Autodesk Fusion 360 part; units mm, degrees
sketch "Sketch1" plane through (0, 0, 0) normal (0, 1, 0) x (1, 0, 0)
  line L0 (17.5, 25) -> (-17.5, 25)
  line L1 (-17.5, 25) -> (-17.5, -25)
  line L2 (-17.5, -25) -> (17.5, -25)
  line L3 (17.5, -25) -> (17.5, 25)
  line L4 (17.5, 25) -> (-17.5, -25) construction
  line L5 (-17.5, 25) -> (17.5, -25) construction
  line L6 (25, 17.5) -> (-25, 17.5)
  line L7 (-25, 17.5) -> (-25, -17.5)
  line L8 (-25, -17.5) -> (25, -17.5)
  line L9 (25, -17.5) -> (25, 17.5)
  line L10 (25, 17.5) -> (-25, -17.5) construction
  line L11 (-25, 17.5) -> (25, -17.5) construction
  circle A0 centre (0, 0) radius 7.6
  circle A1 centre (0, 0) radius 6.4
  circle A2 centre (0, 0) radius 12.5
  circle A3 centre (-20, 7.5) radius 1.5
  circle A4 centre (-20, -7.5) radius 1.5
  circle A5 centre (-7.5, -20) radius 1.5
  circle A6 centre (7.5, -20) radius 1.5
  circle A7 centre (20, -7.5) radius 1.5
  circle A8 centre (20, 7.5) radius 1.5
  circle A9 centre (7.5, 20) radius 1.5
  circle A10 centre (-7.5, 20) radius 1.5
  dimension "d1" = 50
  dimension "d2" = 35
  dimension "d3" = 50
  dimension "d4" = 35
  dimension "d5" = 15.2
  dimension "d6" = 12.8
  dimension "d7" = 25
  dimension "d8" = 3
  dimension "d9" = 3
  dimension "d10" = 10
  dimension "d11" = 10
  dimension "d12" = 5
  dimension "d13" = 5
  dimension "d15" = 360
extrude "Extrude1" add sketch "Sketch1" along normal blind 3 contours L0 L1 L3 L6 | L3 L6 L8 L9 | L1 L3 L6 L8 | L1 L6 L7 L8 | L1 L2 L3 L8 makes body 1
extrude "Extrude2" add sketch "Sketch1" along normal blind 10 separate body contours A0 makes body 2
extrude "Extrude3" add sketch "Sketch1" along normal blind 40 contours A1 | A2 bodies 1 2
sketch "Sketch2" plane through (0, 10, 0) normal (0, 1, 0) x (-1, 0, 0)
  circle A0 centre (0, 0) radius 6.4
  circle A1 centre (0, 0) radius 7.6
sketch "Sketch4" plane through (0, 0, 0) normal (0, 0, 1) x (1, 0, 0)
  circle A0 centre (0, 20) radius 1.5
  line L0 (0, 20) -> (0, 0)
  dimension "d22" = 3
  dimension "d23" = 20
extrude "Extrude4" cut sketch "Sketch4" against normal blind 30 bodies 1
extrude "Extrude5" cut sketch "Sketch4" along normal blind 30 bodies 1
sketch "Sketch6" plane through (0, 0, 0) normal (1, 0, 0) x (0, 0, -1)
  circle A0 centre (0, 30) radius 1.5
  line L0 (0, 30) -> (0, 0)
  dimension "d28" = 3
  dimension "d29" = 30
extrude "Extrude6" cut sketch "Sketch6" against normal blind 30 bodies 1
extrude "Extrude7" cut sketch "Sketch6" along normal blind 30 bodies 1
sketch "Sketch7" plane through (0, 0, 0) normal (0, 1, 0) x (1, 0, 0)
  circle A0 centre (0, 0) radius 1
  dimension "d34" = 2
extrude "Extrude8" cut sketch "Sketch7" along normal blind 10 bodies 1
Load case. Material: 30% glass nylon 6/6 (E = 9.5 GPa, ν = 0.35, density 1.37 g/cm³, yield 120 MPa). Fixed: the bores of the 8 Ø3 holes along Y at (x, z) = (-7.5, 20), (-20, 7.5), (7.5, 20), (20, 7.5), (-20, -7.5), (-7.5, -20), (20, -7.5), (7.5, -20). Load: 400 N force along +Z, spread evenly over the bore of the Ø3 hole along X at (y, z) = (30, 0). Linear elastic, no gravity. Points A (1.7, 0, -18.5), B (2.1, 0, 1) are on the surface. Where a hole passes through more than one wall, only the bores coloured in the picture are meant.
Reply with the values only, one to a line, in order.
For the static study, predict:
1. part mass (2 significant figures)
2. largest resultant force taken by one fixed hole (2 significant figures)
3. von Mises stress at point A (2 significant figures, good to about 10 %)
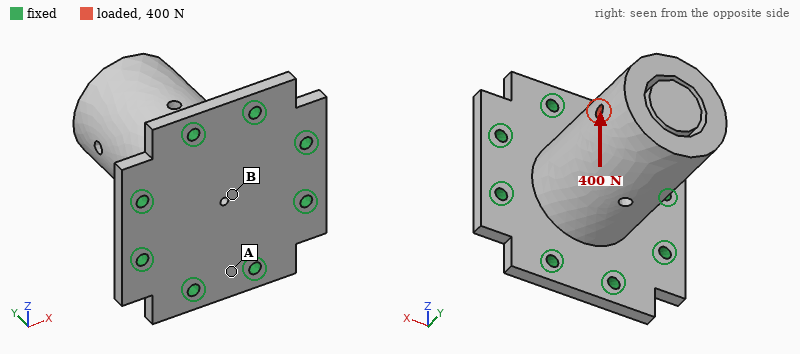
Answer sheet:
31 g
180 N
10 MPa
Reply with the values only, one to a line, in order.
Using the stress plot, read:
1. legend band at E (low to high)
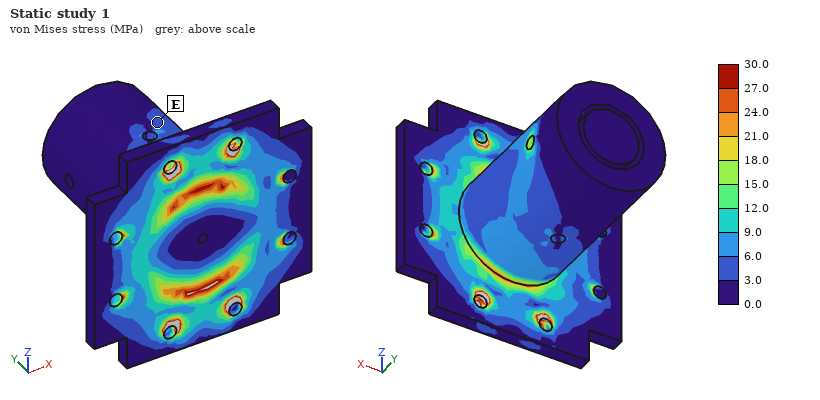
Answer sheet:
3.0 to 6.0 MPa
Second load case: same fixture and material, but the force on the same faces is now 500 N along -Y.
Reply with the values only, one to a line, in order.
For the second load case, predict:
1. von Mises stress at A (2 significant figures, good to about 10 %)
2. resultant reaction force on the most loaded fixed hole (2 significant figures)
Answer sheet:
6.2 MPa
130 N
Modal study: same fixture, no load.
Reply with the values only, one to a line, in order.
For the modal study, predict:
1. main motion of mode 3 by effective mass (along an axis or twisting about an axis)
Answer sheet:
along Y
